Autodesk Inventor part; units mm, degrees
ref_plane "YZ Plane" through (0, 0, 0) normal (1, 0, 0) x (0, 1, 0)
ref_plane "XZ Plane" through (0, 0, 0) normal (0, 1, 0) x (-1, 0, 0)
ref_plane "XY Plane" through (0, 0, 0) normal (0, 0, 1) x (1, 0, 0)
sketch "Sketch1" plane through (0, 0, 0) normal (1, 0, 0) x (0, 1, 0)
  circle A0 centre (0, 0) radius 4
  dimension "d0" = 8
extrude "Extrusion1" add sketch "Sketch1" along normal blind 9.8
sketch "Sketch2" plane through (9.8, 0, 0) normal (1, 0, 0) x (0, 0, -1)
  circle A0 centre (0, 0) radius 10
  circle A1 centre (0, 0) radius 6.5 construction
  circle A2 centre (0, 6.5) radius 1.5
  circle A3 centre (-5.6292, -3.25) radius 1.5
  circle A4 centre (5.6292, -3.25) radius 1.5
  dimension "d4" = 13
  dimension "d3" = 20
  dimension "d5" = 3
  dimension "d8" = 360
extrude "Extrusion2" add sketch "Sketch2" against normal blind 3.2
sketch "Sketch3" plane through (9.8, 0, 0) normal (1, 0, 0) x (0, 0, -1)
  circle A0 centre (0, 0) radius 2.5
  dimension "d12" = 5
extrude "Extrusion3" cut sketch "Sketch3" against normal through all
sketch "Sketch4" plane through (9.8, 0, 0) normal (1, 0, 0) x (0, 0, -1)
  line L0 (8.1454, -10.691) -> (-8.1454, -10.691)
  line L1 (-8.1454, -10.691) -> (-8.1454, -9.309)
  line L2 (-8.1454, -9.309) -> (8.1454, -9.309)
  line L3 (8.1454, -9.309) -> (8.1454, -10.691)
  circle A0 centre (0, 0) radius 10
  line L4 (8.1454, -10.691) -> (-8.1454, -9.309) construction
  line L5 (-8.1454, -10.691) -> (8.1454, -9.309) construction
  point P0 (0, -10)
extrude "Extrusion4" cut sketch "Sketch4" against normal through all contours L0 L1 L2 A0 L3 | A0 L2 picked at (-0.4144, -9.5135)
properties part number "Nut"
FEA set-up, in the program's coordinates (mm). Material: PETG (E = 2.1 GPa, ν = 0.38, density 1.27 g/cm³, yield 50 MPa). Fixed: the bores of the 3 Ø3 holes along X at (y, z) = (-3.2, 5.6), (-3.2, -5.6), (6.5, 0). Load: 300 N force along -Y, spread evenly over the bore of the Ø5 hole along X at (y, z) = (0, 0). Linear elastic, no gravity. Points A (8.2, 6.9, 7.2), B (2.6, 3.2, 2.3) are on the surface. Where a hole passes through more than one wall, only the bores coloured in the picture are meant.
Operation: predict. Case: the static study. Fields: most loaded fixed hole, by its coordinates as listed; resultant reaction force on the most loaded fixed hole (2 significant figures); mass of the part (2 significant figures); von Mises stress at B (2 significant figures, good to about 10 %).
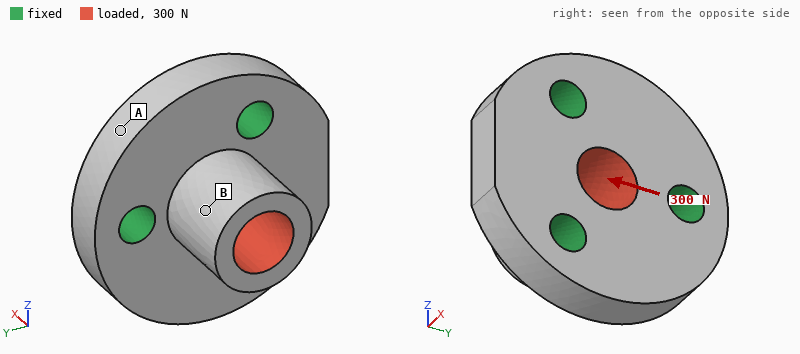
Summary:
(6.5, 0)
150 N
1.4 g
5.1 MPa
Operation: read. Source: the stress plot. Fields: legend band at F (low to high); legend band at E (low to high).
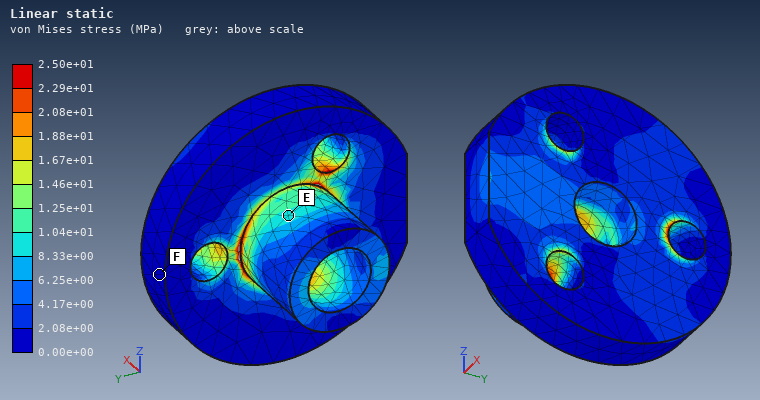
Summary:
0.00e+00 to 2.08e+00 MPa
8.33e+00 to 1.04e+01 MPa
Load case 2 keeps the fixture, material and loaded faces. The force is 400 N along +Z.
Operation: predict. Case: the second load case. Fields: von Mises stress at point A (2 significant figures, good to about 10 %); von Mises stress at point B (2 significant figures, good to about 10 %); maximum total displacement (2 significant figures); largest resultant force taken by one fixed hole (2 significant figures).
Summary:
2.7 MPa
8.7 MPa
0.17 mm
180 N
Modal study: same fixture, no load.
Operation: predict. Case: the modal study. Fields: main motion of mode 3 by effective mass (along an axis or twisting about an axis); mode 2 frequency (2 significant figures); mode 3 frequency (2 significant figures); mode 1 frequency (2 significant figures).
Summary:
along X
14 kHz
17 kHz
14 kHz
